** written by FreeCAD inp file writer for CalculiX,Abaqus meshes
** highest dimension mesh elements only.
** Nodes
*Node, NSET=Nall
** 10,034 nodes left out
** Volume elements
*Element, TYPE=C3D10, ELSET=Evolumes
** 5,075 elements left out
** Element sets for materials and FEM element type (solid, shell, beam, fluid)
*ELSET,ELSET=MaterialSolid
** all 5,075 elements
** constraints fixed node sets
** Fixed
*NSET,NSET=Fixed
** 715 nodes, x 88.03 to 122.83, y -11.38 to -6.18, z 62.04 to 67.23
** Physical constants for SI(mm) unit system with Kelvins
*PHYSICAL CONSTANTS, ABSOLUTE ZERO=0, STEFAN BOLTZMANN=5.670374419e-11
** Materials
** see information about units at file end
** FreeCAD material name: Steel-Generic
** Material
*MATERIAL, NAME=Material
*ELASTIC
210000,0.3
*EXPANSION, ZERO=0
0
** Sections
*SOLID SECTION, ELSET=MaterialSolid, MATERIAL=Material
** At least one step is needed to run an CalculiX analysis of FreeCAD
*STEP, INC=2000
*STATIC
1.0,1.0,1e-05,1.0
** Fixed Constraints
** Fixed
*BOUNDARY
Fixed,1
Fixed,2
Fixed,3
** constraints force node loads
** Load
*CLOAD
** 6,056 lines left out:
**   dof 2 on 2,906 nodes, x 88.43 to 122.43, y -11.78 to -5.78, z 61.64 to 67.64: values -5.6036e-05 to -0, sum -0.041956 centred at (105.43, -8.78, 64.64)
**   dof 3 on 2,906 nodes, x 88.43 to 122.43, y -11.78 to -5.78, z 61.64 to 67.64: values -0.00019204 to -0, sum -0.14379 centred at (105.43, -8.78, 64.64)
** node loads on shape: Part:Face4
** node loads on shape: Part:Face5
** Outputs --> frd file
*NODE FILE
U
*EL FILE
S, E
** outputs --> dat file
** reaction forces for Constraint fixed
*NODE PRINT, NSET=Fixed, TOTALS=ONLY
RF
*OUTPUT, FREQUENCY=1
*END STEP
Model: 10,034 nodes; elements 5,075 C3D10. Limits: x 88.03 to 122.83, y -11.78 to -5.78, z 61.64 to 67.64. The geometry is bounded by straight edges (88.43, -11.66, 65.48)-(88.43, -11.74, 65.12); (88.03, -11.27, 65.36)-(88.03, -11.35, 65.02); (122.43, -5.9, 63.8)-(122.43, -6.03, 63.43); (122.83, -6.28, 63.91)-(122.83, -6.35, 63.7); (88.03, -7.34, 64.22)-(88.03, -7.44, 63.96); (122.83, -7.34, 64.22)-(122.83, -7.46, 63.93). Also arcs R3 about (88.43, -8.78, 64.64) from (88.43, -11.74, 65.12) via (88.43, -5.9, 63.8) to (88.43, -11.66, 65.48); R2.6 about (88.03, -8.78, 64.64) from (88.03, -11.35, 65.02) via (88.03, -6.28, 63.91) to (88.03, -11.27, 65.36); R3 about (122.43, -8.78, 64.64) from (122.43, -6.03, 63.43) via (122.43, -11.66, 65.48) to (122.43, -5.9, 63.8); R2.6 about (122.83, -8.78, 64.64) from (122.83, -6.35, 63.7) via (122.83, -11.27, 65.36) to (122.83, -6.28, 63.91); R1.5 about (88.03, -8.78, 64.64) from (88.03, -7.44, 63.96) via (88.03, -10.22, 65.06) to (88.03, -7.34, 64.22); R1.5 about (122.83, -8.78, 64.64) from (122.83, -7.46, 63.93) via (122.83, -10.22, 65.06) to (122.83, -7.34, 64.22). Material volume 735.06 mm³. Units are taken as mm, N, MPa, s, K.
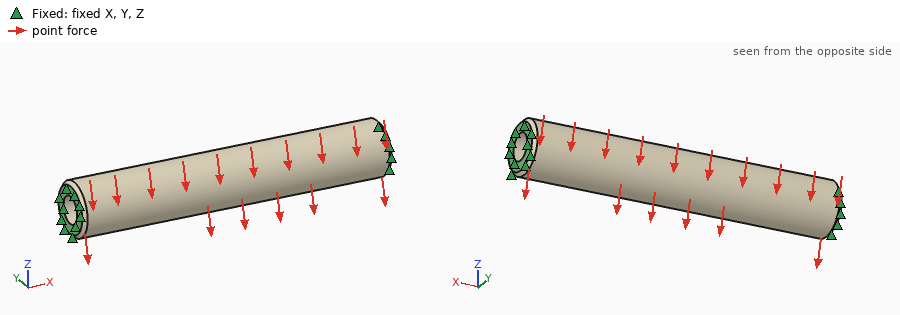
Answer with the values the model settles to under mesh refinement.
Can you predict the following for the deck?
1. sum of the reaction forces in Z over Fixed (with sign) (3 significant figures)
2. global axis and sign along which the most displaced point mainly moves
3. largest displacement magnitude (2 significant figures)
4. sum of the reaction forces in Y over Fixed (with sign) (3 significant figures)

0.144 N
-Z
2.1e-06 mm
0.0420 N
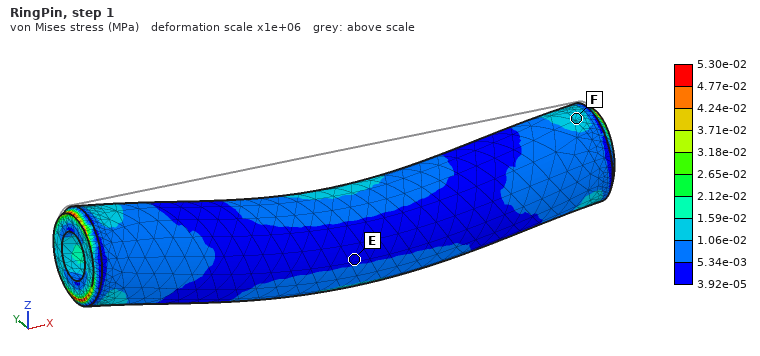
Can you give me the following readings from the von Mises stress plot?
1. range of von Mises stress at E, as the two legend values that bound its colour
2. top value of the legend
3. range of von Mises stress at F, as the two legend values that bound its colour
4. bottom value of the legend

3.92e-05 to 5.34e-03 MPa
5.30e-02 MPa
1.06e-02 to 1.59e-02 MPa
3.92e-05 MPa
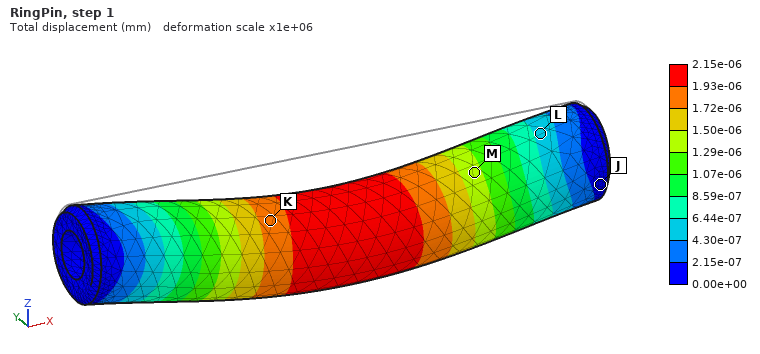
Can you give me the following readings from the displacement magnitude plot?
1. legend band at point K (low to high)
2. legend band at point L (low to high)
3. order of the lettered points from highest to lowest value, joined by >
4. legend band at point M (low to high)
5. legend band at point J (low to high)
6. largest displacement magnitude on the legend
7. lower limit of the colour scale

1.72e-06 to 1.93e-06 mm
4.30e-07 to 6.44e-07 mm
K > M > L > J
1.29e-06 to 1.50e-06 mm
0.00e+00 to 2.15e-07 mm
2.15e-06 mm
0.00e+00 mm
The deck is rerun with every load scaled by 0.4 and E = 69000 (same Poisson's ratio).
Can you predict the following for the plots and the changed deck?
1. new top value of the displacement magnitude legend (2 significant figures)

2.6e-06 mm
